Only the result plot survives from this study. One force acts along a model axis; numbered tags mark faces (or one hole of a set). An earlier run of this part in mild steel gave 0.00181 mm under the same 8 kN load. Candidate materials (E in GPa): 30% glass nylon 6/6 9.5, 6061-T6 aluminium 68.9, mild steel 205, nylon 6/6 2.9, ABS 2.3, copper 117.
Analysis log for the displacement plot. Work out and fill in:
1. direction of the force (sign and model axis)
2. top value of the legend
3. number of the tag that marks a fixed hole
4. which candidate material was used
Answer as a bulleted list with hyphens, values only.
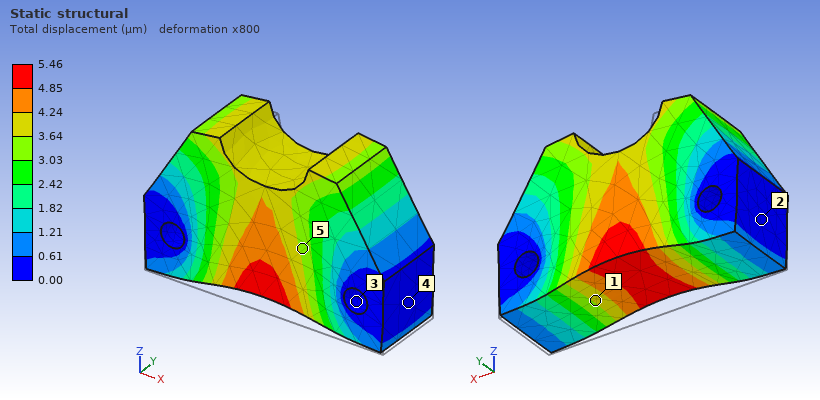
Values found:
- +Z
- 5.46 µm
- 3
- 6061-T6 aluminium
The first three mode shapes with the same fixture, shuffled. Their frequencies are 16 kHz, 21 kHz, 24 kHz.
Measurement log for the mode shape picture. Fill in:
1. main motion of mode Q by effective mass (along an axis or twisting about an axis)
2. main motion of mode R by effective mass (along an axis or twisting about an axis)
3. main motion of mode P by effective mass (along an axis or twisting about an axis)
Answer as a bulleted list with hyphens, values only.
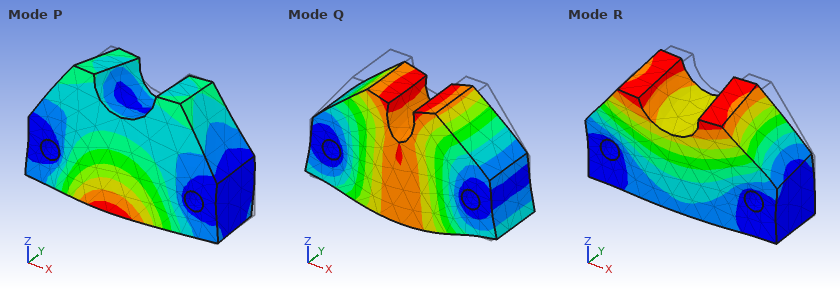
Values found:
- along Z
- along Y
- along Y
